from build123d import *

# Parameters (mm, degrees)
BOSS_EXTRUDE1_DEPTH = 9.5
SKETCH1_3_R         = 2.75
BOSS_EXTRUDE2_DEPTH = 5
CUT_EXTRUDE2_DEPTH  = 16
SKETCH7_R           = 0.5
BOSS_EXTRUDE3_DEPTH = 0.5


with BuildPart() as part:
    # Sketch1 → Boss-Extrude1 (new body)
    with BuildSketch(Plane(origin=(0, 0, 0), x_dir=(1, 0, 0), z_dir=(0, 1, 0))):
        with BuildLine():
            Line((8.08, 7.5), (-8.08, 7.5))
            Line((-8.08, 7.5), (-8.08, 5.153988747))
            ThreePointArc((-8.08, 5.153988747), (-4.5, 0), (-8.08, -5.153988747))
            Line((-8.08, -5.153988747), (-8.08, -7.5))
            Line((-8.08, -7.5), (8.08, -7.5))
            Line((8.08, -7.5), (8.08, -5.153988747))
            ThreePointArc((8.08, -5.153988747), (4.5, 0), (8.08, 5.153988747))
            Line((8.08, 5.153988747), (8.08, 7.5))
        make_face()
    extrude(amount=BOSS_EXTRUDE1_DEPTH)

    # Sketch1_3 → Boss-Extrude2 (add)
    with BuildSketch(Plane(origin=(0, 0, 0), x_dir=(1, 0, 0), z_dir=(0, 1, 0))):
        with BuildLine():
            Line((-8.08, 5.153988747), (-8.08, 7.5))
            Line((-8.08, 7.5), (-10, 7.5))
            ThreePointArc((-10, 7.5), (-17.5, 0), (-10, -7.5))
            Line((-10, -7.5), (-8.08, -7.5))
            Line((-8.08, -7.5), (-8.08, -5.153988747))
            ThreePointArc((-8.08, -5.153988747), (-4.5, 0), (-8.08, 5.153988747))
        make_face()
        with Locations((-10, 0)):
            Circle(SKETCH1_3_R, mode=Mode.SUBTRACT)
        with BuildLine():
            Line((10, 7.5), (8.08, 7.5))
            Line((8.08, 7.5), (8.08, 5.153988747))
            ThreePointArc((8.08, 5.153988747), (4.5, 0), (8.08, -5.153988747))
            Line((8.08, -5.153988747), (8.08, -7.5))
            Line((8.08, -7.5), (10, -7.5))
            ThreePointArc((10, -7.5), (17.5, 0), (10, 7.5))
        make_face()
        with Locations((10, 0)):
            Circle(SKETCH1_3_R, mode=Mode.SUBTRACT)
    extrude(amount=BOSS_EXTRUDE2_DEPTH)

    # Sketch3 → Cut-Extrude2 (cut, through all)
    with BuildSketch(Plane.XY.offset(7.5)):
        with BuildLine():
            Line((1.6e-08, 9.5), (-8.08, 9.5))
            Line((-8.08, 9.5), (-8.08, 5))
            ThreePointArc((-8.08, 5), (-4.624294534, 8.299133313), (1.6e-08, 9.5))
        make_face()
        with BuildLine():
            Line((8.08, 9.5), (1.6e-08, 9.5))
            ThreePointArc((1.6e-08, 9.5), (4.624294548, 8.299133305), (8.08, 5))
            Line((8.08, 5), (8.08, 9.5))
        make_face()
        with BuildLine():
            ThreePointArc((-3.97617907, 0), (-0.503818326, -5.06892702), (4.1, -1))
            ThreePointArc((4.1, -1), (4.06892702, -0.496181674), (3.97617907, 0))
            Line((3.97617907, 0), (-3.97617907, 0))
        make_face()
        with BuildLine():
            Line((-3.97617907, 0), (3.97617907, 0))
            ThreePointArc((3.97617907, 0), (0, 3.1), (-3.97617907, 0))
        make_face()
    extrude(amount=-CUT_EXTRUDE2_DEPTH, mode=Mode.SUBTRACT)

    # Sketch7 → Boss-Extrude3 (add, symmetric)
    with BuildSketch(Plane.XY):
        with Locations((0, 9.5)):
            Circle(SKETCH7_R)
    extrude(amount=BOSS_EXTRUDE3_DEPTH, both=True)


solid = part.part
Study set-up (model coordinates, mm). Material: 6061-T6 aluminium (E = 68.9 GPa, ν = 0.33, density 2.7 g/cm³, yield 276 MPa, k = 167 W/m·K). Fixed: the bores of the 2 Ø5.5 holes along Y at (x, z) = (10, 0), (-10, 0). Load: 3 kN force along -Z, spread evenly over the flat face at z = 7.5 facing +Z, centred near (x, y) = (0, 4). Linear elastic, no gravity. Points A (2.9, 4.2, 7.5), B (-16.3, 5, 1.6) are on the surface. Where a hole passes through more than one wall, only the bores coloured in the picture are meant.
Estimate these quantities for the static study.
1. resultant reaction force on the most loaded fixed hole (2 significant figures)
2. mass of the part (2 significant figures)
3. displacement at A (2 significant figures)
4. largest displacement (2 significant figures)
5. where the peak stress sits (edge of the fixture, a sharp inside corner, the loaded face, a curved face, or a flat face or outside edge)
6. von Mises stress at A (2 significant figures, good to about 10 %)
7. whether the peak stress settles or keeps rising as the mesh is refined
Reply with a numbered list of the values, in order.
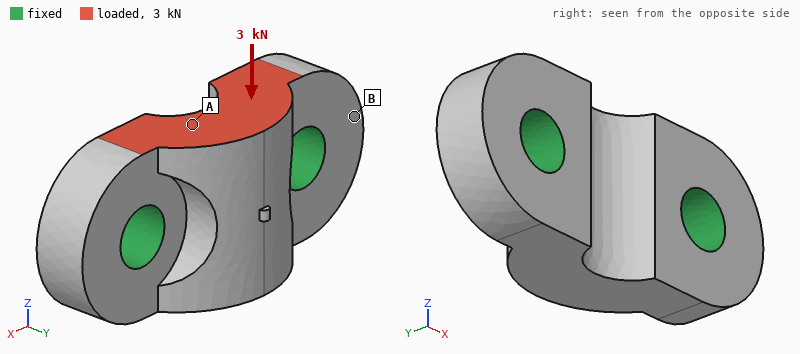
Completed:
1. 1.5 kN
2. 6.9 g
3. 9.8 µm
4. 15 µm
5. edge of the fixture
6. 33 MPa
7. keeps rising
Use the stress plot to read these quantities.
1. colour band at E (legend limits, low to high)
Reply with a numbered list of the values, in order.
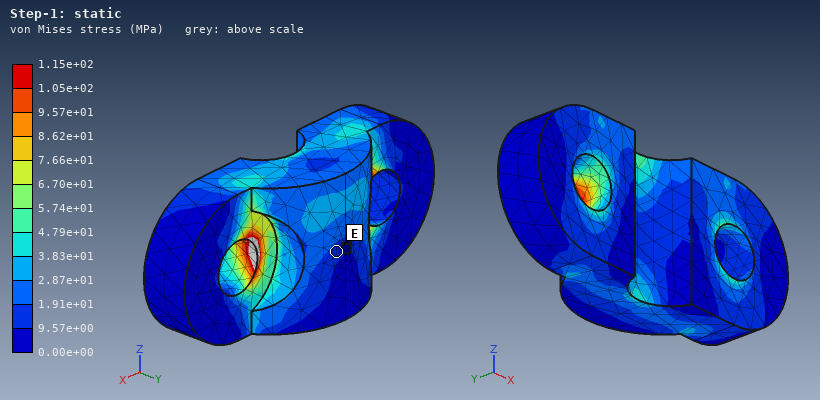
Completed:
1. 9.57e+00 to 1.91e+01 MPa
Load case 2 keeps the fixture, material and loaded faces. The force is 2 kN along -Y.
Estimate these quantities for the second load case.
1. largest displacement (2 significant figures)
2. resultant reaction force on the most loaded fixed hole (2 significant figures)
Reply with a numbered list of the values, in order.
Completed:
1. 25 µm
2. 1.1 kN
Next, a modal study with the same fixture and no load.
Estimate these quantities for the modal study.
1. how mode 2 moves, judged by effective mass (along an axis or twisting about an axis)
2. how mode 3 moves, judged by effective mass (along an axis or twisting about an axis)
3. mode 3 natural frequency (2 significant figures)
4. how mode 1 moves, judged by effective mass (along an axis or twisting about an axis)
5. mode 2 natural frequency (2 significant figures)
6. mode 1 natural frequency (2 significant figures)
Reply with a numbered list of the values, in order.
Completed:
1. along Y
2. along Z
3. 73 kHz
4. along Z
5. 55 kHz
6. 38 kHz
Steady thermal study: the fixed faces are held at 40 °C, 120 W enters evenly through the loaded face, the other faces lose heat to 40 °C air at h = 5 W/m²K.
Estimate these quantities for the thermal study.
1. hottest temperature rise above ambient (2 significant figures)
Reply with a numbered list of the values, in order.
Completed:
1. 52 K
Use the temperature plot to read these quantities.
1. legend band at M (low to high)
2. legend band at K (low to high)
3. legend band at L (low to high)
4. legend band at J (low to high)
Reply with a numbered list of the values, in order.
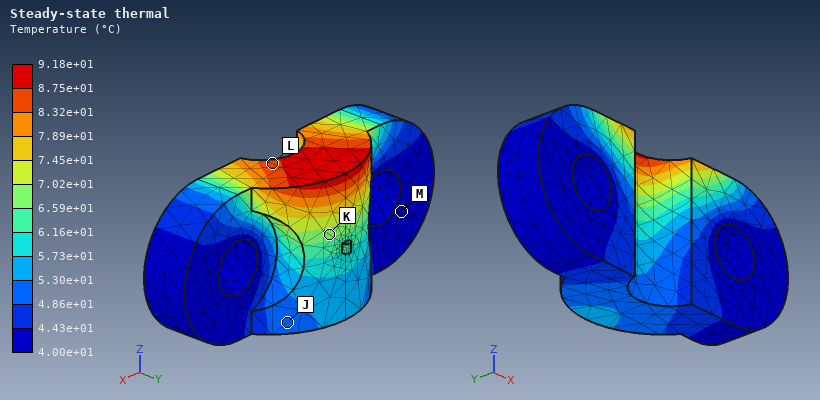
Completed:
1. 4.00e+01 to 4.43e+01 °C
2. 6.59e+01 to 7.02e+01 °C
3. 8.32e+01 to 8.75e+01 °C
4. 4.86e+01 to 5.30e+01 °C
